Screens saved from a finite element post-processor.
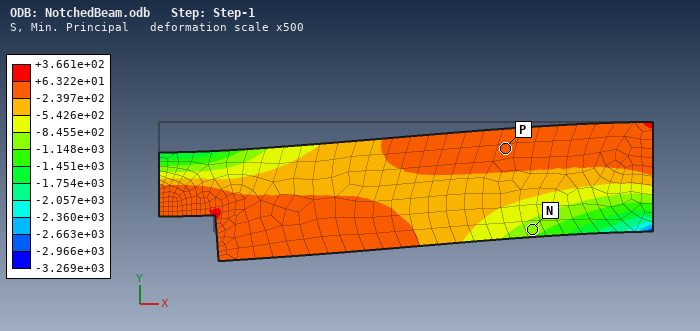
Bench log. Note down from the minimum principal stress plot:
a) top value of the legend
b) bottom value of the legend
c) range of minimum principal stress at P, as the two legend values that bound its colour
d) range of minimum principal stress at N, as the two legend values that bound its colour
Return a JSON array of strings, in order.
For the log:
["+3.661e+02", "-3.269e+03", "-2.397e+02 to +6.322e+01", "-1.148e+03 to -8.455e+02"]
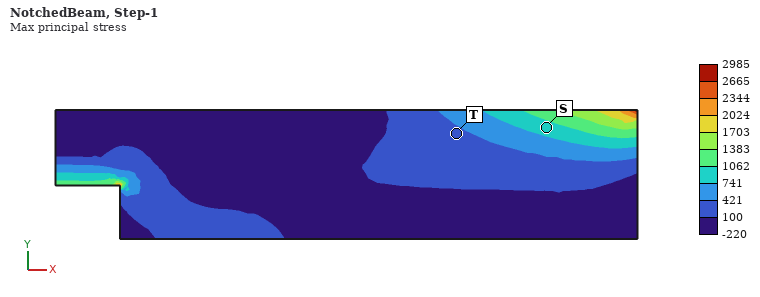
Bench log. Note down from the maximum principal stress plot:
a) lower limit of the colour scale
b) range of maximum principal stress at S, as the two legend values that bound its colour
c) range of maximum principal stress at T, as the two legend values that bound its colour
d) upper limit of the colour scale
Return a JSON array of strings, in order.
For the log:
["-220", "741 to 1062", "100 to 421", "2985"]
